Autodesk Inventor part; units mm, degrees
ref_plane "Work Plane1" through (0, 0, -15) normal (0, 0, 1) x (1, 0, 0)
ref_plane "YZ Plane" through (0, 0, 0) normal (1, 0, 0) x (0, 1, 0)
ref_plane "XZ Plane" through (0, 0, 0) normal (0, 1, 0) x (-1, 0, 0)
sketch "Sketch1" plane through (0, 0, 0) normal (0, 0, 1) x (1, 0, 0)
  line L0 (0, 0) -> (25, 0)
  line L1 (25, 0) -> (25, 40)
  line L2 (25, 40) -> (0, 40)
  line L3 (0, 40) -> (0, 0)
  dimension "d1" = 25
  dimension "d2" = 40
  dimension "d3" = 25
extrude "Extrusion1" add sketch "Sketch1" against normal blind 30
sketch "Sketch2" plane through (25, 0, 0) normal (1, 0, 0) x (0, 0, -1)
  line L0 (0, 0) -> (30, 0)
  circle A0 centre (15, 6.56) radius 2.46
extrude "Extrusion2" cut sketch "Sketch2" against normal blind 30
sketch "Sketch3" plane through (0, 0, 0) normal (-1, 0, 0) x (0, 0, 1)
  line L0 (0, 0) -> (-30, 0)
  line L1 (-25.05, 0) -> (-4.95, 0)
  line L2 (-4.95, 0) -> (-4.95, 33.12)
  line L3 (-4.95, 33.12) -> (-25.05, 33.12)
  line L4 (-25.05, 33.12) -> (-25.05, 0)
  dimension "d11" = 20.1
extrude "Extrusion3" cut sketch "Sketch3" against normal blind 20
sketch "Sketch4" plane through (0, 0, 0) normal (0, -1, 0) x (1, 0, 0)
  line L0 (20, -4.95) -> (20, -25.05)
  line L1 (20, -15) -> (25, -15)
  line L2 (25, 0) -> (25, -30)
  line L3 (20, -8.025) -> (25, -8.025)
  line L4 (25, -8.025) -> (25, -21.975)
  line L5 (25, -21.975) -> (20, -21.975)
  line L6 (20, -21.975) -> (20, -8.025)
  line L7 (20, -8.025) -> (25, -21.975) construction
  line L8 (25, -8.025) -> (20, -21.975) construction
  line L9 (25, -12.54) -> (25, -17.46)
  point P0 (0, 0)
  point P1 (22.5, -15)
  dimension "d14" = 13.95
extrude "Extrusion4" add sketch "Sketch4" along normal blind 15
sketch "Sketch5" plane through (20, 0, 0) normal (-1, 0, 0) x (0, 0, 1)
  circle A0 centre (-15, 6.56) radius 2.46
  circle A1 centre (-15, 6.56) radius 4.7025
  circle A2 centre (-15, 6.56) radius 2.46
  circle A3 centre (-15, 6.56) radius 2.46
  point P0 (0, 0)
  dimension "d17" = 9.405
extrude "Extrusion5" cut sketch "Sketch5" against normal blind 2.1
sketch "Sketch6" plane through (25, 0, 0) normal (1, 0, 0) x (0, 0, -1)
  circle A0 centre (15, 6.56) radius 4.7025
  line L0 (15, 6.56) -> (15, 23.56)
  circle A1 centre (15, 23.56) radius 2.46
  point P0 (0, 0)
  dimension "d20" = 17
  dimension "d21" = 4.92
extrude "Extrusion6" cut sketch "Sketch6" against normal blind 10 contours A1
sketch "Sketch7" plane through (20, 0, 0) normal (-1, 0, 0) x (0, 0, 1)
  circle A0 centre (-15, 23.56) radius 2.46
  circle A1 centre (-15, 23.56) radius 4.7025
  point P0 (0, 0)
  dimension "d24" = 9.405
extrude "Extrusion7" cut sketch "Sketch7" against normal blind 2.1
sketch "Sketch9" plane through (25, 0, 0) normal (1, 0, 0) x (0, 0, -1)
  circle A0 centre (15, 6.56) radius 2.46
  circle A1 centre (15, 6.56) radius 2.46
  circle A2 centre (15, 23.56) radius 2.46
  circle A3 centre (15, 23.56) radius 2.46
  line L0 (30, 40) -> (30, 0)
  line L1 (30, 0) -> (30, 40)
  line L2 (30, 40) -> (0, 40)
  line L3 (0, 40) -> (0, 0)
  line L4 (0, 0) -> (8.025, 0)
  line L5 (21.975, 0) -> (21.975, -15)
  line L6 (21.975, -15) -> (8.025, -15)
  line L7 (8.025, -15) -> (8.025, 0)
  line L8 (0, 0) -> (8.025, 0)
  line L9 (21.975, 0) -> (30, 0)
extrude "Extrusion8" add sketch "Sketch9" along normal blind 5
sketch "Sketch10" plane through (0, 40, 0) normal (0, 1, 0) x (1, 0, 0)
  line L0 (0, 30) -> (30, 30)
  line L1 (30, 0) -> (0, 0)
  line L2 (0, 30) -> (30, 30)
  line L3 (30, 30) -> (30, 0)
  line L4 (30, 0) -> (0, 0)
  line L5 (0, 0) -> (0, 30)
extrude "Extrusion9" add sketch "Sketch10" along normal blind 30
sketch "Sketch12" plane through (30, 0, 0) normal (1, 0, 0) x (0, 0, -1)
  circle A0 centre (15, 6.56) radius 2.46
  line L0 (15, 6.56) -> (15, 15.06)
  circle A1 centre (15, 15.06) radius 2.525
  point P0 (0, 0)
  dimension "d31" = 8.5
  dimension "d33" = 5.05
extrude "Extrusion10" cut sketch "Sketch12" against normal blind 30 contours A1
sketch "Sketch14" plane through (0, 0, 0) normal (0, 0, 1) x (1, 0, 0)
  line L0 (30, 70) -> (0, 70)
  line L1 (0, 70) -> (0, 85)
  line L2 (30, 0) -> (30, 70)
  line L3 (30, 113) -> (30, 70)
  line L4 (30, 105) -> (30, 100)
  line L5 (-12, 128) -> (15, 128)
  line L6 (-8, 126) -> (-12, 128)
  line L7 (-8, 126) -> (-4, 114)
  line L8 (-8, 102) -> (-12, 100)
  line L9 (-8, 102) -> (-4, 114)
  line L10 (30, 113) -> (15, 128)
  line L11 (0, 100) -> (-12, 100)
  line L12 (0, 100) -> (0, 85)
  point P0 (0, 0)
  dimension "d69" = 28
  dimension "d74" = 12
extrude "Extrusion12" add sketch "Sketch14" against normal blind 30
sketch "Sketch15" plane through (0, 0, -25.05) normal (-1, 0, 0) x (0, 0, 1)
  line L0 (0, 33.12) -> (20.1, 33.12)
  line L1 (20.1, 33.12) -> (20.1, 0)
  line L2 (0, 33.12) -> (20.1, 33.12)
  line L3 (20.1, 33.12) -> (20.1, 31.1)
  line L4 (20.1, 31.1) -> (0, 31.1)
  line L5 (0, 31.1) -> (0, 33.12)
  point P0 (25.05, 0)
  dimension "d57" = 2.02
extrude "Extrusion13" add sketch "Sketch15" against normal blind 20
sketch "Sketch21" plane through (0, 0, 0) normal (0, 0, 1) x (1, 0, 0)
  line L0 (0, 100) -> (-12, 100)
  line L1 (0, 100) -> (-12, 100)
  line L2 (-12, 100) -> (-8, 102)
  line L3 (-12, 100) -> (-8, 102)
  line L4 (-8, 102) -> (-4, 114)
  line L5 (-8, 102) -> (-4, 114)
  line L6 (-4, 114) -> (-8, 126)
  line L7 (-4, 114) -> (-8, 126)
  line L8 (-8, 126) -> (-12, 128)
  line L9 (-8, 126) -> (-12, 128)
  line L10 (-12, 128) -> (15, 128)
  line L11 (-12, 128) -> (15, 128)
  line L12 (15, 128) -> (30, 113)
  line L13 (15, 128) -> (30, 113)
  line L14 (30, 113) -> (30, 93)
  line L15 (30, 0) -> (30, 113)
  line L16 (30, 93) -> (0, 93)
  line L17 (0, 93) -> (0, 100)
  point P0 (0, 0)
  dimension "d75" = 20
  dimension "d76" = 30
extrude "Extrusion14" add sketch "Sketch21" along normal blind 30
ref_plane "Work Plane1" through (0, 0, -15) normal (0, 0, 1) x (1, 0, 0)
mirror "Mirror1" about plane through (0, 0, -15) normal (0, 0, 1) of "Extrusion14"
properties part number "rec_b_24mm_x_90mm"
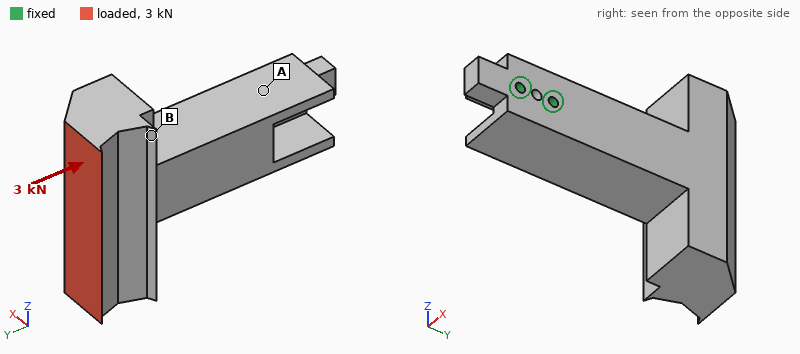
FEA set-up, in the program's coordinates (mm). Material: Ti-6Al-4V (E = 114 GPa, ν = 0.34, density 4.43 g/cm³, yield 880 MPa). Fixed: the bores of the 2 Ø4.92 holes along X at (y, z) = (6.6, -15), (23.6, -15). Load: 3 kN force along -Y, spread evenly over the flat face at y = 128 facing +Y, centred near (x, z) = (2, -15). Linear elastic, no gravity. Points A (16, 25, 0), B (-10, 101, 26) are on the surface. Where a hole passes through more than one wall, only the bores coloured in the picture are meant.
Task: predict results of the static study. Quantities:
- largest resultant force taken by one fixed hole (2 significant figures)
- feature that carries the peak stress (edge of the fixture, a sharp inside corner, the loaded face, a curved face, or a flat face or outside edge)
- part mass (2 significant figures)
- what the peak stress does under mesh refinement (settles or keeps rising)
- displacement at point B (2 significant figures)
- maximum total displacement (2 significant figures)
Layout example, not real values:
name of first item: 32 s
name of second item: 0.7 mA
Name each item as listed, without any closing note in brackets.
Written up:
largest resultant force taken by one fixed hole: 3.4 kN
feature that carries the peak stress: edge of the fixture
part mass: 770 g
what the peak stress does under mesh refinement: keeps rising
displacement at point B: 0.098 mm
maximum total displacement: 0.13 mm
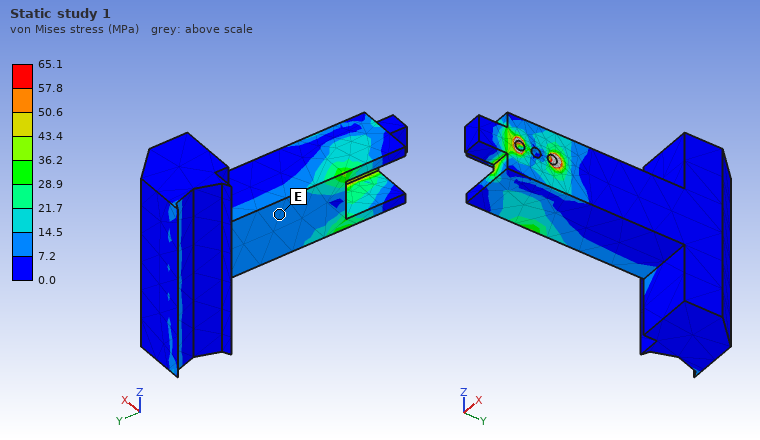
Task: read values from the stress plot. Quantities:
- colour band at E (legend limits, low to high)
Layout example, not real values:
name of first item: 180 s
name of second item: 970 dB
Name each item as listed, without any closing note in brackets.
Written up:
colour band at E: 7.2 to 14.5 MPa
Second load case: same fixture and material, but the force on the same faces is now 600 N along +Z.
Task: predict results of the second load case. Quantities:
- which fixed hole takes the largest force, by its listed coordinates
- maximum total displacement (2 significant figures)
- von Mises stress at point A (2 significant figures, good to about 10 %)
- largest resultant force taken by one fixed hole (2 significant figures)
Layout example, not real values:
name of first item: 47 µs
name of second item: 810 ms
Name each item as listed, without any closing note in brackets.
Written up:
which fixed hole takes the largest force, by its listed coordinates: (23.6, -15)
maximum total displacement: 0.10 mm
von Mises stress at point A: 22 MPa
largest resultant force taken by one fixed hole: 3.3 kN
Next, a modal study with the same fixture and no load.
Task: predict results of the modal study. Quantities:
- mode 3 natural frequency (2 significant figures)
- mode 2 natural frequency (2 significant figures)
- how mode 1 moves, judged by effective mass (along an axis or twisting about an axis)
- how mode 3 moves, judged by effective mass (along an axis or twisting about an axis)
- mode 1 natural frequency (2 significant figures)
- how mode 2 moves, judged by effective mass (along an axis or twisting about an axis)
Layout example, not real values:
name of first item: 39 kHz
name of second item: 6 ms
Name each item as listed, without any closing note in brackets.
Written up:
mode 3 natural frequency: 1300 Hz
mode 2 natural frequency: 700 Hz
how mode 1 moves, judged by effective mass: along X
how mode 3 moves, judged by effective mass: twisting about Y
mode 1 natural frequency: 620 Hz
how mode 2 moves, judged by effective mass: along Z
